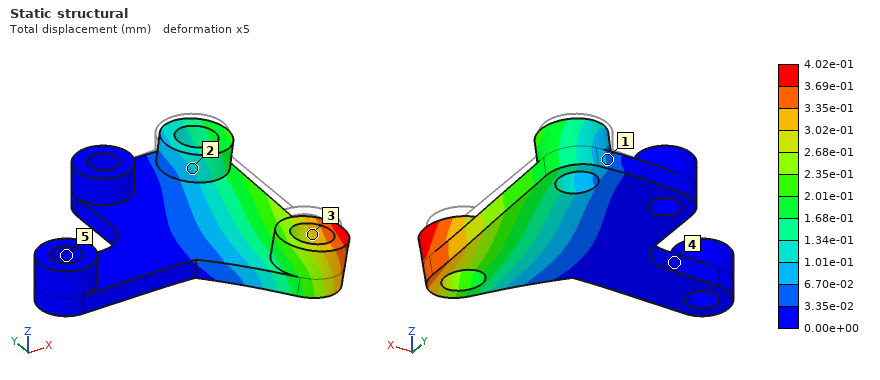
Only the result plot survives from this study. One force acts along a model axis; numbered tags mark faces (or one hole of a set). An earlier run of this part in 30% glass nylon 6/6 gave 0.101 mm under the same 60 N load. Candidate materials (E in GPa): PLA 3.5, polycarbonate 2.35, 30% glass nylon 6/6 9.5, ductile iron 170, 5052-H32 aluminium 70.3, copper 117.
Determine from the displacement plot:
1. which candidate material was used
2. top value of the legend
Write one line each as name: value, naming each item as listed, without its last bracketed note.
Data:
which candidate material was used: polycarbonate
top value of the legend: 4.02e-01 mm
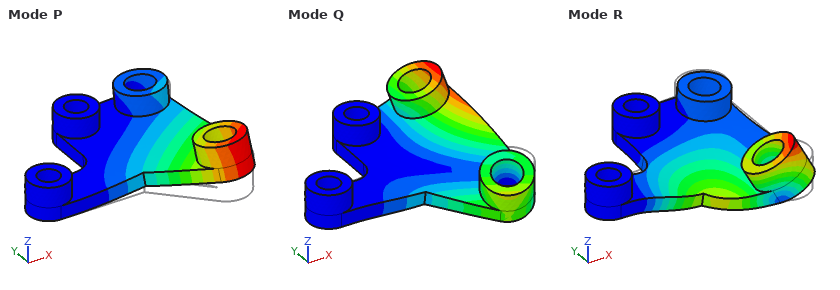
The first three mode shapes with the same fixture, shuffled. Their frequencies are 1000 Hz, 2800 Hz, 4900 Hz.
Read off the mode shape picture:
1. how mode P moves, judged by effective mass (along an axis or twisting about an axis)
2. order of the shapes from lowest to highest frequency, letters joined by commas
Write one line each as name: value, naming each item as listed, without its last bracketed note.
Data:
how mode P moves, judged by effective mass: along Z
order of the shapes from lowest to highest frequency, letters joined by commas: P, Q, R
